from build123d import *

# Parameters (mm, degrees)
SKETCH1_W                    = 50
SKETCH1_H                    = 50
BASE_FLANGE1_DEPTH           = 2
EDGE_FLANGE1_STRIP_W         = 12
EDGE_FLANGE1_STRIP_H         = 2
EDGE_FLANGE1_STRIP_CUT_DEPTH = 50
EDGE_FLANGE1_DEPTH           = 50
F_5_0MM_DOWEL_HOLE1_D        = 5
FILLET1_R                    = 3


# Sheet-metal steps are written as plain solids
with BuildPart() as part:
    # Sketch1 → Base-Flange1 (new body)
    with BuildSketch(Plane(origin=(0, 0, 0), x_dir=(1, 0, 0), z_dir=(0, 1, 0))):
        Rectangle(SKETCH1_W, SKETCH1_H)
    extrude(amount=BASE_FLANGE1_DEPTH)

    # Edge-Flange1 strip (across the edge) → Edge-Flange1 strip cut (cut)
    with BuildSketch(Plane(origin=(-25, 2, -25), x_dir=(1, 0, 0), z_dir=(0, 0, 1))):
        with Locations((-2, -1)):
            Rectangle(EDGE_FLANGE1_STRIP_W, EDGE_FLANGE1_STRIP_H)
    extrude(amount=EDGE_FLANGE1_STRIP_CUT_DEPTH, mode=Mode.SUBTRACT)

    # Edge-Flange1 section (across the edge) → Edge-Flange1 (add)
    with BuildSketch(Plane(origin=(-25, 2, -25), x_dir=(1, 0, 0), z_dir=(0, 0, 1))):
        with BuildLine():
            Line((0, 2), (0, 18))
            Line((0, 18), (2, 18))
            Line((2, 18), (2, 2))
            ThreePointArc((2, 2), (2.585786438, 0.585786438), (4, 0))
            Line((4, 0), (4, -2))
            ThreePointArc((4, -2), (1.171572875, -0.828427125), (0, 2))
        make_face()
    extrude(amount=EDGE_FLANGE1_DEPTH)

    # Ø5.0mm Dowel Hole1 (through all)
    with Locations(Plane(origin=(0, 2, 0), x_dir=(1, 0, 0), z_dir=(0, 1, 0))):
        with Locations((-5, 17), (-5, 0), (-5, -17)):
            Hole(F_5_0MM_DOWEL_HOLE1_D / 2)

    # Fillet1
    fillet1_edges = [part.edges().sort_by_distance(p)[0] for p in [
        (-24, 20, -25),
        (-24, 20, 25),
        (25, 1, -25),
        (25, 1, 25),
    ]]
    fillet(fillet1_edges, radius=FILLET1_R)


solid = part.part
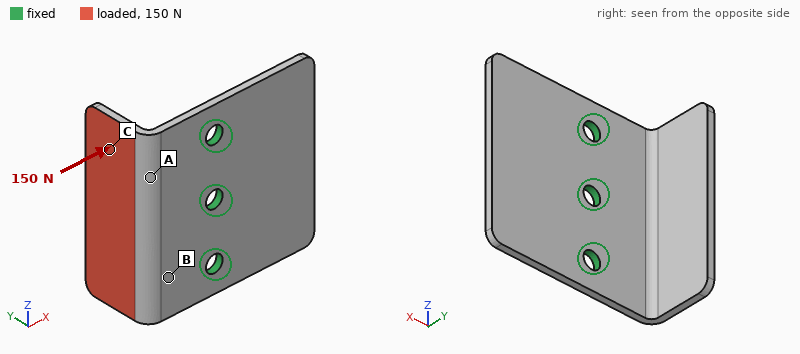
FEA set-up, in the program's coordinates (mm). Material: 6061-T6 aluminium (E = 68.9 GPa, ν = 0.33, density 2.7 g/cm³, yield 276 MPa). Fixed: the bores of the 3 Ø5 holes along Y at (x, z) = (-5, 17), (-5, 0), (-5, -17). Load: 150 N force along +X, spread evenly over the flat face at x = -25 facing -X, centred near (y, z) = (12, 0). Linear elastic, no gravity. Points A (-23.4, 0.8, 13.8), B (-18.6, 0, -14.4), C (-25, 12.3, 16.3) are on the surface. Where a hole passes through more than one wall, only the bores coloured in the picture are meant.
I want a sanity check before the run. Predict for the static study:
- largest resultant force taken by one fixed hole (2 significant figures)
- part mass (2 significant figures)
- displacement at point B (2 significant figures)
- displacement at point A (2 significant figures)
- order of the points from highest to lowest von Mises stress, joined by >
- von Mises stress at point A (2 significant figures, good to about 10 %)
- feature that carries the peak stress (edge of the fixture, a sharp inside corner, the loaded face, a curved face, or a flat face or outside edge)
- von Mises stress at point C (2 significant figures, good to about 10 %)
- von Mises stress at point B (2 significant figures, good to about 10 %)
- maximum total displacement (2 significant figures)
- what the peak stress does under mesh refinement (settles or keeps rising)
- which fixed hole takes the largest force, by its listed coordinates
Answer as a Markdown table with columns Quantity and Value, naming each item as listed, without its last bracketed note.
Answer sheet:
| Quantity | Value |
|---|---|
| largest resultant force taken by one fixed hole | 55 N |
| part mass | 18 g |
| displacement at point B | 0.051 mm |
| displacement at point A | 0.096 mm |
| order of the points from highest to lowest von Mises stress, joined by > | B > A > C |
| von Mises stress at point A | 34 MPa |
| feature that carries the peak stress | edge of the fixture |
| von Mises stress at point C | 7.4 MPa |
| von Mises stress at point B | 42 MPa |
| maximum total displacement | 0.29 mm |
| what the peak stress does under mesh refinement | keeps rising |
| which fixed hole takes the largest force, by its listed coordinates | (-5, 0) |
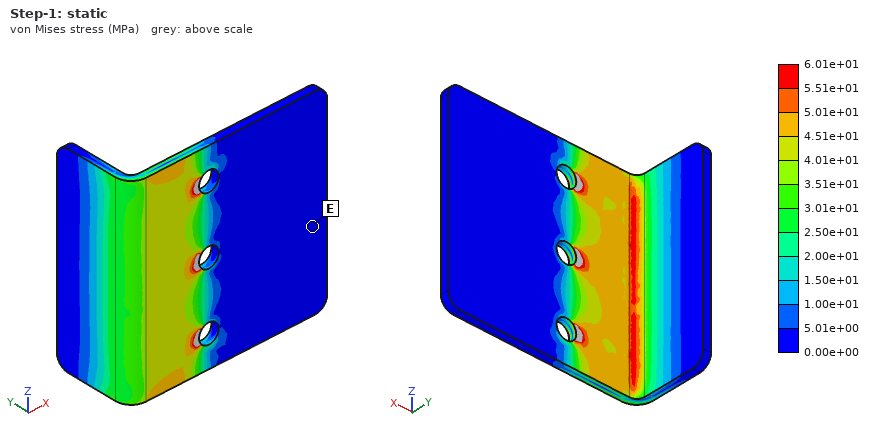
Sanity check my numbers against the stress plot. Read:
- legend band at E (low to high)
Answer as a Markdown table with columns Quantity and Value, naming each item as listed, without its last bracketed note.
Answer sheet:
| Quantity | Value |
|---|---|
| legend band at E | 0.00e+00 to 5.01e+00 MPa |
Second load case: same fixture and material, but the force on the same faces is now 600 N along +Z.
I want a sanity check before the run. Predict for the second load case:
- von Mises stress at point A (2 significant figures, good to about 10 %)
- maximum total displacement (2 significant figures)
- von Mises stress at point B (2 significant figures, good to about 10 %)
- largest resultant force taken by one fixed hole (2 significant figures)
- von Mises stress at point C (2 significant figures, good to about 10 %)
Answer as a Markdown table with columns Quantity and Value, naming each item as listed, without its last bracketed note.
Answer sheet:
| Quantity | Value |
|---|---|
| von Mises stress at point A | 45 MPa |
| maximum total displacement | 0.31 mm |
| von Mises stress at point B | 49 MPa |
| largest resultant force taken by one fixed hole | 400 N |
| von Mises stress at point C | 20 MPa |
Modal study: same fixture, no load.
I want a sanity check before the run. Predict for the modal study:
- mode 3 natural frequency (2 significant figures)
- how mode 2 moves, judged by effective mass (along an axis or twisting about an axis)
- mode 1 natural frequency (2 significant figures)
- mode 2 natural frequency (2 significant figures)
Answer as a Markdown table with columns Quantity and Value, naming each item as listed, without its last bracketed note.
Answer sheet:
| Quantity | Value |
|---|---|
| mode 3 natural frequency | 2800 Hz |
| how mode 2 moves, judged by effective mass | along Y |
| mode 1 natural frequency | 1700 Hz |
| mode 2 natural frequency | 2100 Hz |
